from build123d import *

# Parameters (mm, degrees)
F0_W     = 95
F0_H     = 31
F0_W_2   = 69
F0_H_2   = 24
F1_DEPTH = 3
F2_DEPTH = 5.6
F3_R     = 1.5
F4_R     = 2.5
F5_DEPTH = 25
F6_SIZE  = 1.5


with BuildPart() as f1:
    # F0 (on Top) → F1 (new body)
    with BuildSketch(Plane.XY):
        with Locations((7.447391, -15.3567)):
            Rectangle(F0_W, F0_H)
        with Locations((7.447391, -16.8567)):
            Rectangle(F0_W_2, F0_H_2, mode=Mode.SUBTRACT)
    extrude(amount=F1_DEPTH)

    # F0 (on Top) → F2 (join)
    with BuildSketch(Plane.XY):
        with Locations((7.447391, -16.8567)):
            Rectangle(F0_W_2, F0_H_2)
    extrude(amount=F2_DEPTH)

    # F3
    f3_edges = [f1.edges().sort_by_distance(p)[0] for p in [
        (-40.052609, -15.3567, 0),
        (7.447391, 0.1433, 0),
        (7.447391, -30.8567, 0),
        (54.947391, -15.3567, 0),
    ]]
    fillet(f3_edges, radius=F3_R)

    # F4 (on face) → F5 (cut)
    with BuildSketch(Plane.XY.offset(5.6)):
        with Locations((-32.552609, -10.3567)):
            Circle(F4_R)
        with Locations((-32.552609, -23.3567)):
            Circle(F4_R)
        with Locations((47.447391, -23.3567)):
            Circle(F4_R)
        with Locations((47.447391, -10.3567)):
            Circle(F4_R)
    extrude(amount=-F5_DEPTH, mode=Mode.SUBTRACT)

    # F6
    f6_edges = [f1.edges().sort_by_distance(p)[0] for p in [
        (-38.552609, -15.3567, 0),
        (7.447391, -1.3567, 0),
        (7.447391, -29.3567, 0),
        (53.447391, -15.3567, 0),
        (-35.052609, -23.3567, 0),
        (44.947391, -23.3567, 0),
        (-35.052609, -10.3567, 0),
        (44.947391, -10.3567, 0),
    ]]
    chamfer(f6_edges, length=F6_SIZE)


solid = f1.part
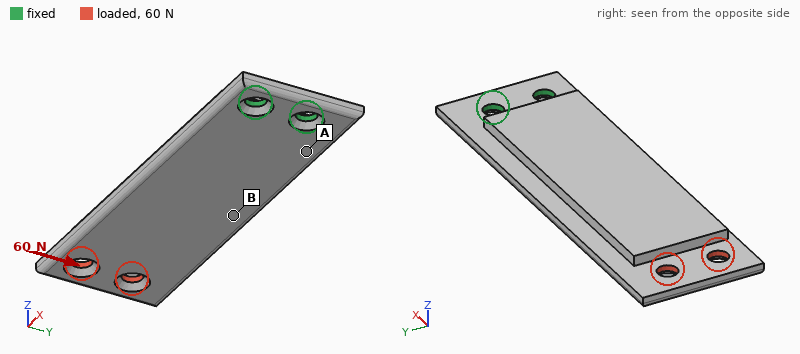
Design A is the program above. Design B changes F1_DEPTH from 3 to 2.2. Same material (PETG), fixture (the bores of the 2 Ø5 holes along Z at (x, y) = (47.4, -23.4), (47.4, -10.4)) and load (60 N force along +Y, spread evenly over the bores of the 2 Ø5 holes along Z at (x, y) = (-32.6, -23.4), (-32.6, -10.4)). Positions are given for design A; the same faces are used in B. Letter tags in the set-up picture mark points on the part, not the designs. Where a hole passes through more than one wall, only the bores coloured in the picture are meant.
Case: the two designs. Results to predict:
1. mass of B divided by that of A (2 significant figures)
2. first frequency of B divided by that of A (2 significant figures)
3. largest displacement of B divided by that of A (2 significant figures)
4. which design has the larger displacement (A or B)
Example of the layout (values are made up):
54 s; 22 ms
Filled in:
0.92; 0.69; 1.3; B
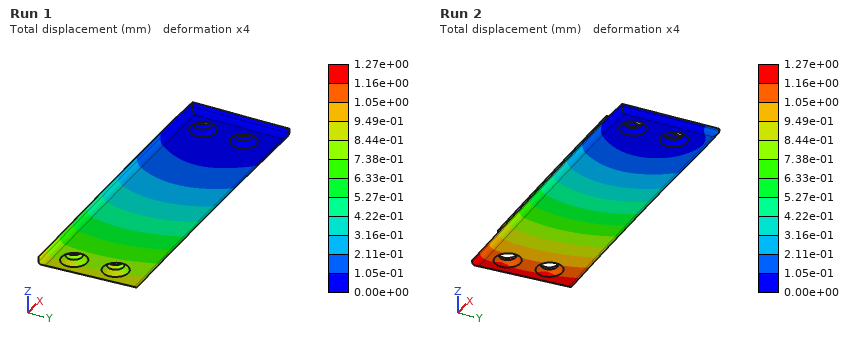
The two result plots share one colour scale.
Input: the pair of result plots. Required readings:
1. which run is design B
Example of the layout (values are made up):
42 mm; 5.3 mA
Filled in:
Run 2
